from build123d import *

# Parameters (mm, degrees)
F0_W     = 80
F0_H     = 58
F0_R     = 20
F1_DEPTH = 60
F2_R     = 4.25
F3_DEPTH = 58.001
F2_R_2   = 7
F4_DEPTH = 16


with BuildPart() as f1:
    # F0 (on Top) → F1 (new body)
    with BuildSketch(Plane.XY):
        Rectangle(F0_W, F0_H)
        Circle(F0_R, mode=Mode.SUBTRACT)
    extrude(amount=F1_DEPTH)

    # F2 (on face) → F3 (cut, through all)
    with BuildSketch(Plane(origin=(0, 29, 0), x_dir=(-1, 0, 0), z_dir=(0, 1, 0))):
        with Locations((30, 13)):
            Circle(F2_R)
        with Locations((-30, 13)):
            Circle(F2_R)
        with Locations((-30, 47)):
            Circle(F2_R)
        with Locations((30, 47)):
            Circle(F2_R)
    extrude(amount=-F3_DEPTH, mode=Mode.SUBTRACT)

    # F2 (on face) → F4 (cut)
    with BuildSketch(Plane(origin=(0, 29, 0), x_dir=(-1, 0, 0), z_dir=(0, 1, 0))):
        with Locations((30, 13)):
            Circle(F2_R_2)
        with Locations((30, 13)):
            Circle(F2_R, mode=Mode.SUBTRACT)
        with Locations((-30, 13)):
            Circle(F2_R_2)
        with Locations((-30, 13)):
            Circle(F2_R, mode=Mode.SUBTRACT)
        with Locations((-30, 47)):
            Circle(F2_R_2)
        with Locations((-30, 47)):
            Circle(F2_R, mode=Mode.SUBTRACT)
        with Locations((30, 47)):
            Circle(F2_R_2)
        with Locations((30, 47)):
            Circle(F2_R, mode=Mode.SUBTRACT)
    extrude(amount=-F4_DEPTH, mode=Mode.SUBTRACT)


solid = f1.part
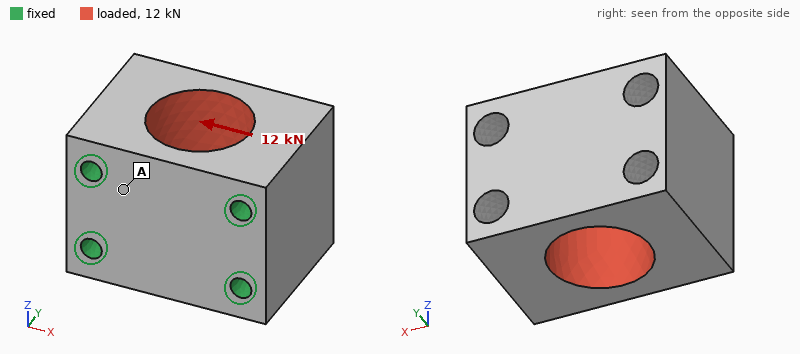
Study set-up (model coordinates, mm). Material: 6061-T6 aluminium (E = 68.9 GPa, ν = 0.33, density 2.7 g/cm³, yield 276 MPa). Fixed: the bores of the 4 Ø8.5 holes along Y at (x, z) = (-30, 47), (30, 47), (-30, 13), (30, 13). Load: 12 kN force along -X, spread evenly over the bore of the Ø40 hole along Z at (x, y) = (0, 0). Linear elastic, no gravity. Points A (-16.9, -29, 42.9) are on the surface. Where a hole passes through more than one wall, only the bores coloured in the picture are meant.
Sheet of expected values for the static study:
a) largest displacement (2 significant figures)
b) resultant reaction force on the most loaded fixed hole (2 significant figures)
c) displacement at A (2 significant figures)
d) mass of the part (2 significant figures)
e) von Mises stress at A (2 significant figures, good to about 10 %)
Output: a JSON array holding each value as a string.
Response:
["2.6 µm", "3.0 kN", "0.40 µm", "500 g", "1.5 MPa"]
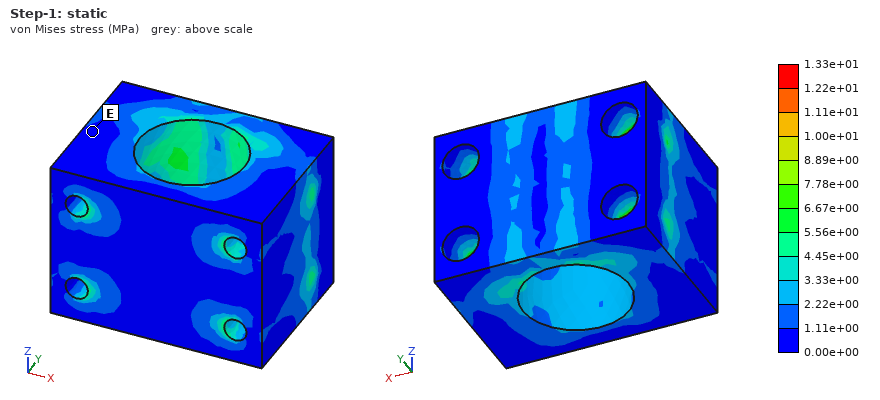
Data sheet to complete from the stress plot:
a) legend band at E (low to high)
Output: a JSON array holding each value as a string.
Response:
["0.00e+00 to 1.11e+00 MPa"]
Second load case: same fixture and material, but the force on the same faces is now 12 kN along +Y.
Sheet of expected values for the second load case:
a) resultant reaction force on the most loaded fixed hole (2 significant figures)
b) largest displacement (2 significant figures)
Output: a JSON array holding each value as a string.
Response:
["3.0 kN", "3.7 µm"]
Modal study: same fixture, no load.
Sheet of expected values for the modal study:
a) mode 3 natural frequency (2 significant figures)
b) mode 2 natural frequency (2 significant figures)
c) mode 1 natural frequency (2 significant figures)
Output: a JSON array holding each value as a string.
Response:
["22 kHz", "18 kHz", "18 kHz"]
